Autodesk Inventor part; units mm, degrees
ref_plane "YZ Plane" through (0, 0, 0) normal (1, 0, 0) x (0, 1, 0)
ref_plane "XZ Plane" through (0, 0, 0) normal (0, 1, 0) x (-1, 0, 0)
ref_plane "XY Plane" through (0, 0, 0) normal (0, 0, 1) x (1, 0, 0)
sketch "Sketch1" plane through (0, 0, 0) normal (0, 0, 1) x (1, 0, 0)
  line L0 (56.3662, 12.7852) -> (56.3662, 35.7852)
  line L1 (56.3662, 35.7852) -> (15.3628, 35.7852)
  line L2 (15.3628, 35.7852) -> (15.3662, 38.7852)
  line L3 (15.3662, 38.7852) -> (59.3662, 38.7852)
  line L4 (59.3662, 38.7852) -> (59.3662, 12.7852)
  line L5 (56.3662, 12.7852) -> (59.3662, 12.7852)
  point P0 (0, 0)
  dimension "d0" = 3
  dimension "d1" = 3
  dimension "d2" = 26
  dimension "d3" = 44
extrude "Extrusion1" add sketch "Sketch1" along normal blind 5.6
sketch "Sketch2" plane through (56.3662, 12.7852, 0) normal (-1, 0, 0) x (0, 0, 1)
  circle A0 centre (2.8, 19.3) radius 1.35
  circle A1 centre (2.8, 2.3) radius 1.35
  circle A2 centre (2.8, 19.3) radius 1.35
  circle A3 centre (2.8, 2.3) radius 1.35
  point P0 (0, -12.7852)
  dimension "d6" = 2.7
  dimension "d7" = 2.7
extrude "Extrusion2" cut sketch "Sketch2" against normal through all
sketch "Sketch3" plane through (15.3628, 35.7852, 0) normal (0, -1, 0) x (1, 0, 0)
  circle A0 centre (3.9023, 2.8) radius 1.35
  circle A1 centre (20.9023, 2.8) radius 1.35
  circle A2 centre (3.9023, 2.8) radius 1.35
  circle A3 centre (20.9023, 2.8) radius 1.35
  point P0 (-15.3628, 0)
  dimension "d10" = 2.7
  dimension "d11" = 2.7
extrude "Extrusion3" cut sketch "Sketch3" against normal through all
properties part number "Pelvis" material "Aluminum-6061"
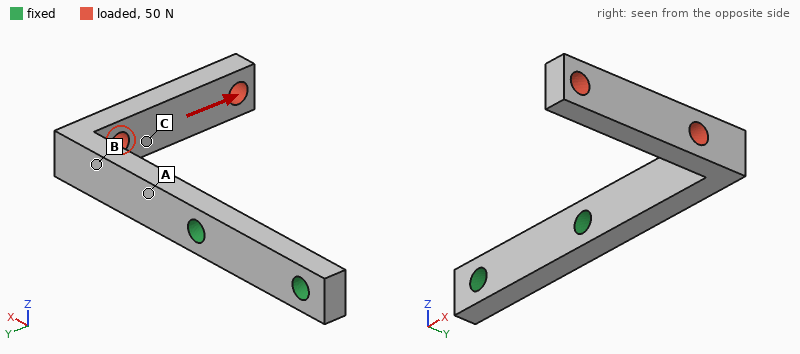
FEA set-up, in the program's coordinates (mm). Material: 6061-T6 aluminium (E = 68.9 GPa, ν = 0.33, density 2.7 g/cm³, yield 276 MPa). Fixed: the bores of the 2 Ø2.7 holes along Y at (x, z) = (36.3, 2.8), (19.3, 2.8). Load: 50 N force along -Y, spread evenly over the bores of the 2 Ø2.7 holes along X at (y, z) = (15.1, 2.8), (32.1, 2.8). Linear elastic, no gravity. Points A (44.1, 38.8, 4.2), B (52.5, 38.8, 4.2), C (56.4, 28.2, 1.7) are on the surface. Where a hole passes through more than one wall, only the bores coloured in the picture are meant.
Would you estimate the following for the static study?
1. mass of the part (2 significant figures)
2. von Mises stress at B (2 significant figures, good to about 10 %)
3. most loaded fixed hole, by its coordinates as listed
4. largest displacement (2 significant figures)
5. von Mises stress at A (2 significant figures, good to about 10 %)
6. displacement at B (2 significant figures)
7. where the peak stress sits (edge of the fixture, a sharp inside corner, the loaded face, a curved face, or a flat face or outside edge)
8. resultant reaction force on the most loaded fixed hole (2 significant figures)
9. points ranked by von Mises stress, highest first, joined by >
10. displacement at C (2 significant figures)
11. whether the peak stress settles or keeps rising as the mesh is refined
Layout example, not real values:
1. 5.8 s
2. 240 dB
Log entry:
1. 2.9 g
2. 32 MPa
3. (36.3, 2.8)
4. 0.36 mm
5. 82 MPa
6. 0.11 mm
7. edge of the fixture
8. 51 N
9. A > B > C
10. 0.19 mm
11. keeps rising
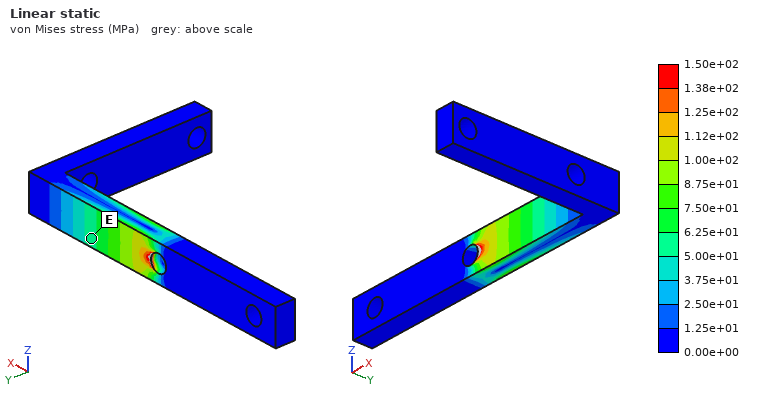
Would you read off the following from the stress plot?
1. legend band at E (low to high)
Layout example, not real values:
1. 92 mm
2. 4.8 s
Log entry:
1. 5.00e+01 to 6.25e+01 MPa
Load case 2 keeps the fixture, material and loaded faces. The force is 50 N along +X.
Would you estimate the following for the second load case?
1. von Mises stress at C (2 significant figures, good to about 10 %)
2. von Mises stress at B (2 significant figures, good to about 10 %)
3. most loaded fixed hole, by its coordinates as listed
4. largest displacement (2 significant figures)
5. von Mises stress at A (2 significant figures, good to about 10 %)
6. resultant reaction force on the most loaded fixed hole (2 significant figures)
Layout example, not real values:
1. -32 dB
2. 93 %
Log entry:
1. 38 MPa
2. 79 MPa
3. (36.3, 2.8)
4. 0.58 mm
5. 79 MPa
6. 49 N
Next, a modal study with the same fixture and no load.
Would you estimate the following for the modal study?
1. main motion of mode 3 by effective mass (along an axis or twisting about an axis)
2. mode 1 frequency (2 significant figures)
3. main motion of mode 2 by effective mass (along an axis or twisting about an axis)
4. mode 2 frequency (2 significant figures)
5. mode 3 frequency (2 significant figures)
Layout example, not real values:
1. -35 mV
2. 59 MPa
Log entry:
1. along Y
2. 1700 Hz
3. along Z
4. 2100 Hz
5. 4400 Hz
